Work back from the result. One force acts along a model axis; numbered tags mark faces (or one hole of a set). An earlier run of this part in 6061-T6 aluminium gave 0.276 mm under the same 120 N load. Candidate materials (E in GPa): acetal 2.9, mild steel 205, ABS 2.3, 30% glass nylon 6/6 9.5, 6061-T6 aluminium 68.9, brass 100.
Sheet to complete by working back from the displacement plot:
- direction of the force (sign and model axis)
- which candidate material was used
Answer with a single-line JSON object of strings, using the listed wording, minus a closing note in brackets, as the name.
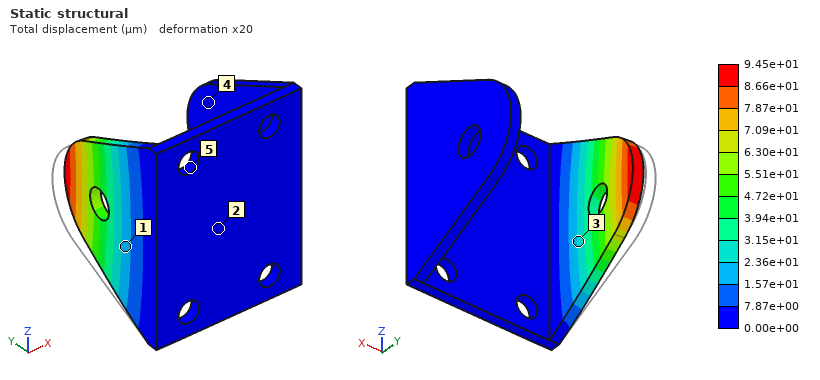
{"direction of the force": "+X", "which candidate material was used": "mild steel"}
